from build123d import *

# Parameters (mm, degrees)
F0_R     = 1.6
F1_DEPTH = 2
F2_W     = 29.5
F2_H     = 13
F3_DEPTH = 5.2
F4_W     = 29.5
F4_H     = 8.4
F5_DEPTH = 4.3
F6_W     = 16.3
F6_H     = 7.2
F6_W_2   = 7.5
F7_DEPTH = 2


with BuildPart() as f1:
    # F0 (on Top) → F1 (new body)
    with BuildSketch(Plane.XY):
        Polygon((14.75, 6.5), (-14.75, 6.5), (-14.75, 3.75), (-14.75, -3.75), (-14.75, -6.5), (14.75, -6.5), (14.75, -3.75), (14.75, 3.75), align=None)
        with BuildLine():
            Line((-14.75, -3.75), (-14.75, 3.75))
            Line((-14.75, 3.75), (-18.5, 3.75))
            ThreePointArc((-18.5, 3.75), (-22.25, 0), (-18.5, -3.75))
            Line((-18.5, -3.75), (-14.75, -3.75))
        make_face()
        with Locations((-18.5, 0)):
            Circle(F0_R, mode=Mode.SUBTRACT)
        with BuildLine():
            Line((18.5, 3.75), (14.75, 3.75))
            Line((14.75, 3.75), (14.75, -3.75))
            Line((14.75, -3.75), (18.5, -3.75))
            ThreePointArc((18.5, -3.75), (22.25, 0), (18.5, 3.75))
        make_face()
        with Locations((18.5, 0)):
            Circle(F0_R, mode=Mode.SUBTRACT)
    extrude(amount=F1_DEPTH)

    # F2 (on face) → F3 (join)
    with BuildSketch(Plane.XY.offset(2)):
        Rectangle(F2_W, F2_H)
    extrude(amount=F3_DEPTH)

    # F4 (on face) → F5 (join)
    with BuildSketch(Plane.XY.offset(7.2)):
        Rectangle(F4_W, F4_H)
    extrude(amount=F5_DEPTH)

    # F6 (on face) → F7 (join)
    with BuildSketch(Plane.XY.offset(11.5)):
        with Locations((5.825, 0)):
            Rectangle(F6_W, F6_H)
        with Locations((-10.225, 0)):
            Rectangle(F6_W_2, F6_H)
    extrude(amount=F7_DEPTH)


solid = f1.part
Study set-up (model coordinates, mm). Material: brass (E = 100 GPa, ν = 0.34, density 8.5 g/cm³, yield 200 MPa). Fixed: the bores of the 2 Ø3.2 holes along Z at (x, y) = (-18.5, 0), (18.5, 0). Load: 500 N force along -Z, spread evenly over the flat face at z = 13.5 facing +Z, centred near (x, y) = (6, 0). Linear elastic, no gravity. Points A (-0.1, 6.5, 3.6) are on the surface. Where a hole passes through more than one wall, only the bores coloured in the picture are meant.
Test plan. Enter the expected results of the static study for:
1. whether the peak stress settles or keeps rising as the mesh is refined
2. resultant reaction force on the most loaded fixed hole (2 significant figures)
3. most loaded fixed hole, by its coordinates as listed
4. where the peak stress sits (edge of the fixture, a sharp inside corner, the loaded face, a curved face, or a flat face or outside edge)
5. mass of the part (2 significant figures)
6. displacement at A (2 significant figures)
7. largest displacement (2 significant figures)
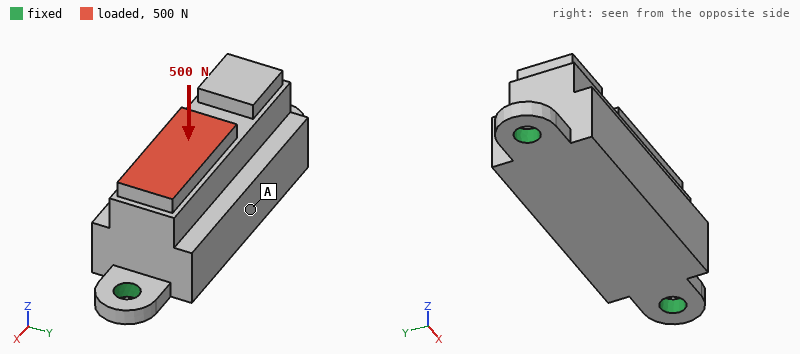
keeps rising
380 N
(18.5, 0)
edge of the fixture
37 g
5.2 µm
5.8 µm
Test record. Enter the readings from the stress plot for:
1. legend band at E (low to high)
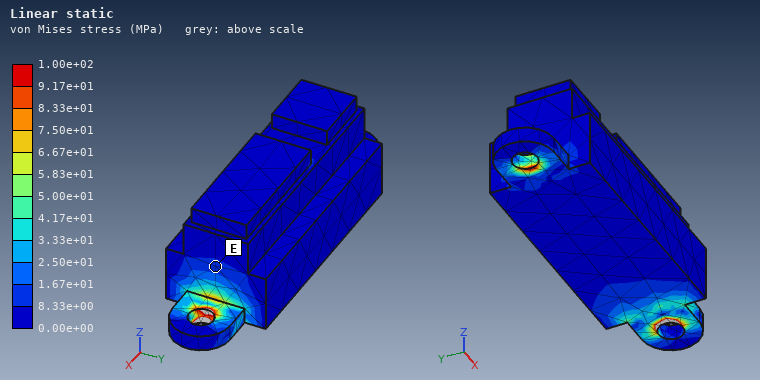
8.33e+00 to 1.67e+01 MPa
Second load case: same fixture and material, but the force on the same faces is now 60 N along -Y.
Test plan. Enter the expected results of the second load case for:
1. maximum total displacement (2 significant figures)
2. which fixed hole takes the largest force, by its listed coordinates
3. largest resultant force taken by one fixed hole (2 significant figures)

17 µm
(18.5, 0)
40 N
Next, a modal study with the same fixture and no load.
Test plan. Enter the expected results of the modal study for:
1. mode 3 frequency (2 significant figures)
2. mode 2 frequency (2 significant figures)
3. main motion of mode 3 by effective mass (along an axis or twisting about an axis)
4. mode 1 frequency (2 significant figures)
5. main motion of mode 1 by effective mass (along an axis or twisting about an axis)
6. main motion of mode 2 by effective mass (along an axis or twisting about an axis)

14 kHz
8700 Hz
along Y
3000 Hz
along Y
along Z
